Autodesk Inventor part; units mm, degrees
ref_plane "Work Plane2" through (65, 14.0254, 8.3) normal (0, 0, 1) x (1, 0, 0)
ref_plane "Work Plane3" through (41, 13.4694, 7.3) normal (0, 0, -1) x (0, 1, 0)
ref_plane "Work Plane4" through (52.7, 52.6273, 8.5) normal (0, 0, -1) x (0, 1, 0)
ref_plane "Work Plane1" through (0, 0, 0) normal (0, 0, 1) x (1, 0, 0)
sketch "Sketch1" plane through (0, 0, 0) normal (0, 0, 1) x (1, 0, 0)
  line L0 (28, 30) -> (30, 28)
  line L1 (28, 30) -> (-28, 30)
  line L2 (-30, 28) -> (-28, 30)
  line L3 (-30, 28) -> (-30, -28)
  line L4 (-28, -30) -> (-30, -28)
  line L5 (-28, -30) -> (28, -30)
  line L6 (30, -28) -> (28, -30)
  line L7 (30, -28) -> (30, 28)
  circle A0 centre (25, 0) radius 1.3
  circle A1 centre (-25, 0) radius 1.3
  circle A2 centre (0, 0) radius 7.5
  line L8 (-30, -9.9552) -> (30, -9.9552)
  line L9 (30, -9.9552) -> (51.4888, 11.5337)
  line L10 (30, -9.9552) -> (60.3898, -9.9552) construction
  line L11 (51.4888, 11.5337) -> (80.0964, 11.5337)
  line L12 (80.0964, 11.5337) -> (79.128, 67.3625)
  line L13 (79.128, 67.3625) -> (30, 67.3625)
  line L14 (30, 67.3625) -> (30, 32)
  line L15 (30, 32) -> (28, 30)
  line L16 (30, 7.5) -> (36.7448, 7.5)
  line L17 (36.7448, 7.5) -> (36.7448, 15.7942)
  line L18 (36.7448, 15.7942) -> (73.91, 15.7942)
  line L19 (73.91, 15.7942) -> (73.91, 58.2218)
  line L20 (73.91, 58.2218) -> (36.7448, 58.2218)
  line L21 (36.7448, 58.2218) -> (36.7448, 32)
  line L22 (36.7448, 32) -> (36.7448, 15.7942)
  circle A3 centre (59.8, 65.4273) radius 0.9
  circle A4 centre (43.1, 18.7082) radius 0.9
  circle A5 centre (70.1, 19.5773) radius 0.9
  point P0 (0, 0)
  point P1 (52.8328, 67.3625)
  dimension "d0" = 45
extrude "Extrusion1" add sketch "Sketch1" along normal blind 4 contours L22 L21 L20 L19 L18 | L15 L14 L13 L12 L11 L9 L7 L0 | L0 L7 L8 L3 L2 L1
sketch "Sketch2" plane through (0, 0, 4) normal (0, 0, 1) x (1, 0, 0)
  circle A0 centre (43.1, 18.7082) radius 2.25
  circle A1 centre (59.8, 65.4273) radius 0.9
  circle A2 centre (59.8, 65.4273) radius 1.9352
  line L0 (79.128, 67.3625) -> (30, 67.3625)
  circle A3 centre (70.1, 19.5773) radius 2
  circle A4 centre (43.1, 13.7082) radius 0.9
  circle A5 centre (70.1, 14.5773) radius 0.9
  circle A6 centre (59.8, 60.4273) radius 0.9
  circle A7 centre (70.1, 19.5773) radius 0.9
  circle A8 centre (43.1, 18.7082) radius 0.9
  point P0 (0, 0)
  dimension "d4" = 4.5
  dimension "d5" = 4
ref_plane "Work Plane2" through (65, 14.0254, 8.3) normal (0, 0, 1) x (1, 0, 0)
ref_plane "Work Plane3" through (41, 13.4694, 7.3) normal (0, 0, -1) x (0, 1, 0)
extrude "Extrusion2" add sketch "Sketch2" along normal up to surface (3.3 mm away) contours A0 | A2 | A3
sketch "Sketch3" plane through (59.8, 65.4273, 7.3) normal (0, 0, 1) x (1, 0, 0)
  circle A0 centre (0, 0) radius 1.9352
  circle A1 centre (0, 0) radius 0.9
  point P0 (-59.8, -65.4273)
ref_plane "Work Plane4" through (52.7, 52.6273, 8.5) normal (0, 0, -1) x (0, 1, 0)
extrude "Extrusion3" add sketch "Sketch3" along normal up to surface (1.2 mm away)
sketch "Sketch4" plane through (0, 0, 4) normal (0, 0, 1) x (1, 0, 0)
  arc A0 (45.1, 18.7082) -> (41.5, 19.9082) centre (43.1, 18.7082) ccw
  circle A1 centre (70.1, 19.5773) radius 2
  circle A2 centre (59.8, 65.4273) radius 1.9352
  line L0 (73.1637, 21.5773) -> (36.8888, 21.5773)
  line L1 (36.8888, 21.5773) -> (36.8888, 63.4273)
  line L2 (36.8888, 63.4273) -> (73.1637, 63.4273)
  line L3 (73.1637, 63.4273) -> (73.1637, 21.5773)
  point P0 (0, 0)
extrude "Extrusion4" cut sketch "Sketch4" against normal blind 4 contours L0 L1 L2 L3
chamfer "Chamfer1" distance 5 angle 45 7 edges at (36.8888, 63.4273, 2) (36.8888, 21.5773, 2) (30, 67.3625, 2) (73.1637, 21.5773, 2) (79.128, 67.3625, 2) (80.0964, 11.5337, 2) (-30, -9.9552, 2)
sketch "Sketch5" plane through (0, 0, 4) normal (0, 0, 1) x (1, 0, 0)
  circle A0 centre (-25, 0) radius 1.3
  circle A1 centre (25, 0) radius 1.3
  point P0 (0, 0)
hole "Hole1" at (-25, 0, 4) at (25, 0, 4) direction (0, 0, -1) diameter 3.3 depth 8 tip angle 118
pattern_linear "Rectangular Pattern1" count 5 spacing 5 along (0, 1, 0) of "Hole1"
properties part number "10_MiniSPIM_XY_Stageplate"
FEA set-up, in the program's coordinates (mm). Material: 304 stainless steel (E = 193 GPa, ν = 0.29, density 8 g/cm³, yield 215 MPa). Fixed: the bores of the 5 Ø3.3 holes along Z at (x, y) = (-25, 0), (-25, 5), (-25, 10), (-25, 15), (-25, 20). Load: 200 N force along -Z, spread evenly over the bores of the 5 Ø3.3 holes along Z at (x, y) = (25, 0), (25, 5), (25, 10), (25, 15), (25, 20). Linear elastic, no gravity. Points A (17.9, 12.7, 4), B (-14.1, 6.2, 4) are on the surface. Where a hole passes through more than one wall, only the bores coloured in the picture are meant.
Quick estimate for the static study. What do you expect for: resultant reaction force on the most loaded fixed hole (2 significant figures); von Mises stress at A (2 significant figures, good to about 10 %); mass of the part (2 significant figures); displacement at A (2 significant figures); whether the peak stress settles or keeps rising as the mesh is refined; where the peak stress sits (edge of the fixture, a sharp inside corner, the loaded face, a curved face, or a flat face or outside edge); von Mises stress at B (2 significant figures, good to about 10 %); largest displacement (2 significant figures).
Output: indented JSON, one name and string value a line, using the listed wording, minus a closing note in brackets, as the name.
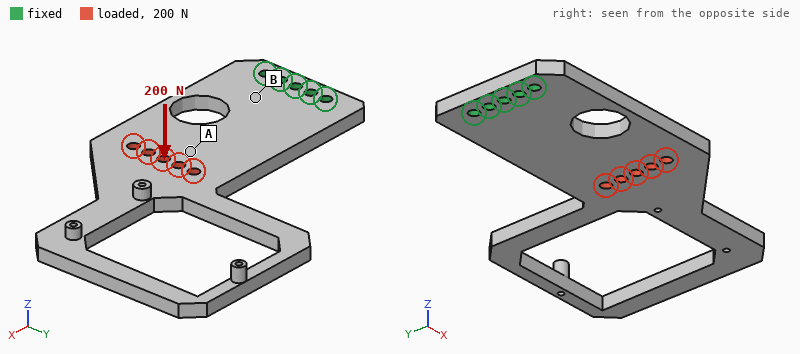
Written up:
{
  "resultant reaction force on the most loaded fixed hole": "89 N",
  "von Mises stress at A": "17 MPa",
  "mass of the part": "120 g",
  "displacement at A": "0.18 mm",
  "whether the peak stress settles or keeps rising as the mesh is refined": "keeps rising",
  "where the peak stress sits": "edge of the fixture",
  "von Mises stress at B": "67 MPa",
  "largest displacement": "0.62 mm"
}
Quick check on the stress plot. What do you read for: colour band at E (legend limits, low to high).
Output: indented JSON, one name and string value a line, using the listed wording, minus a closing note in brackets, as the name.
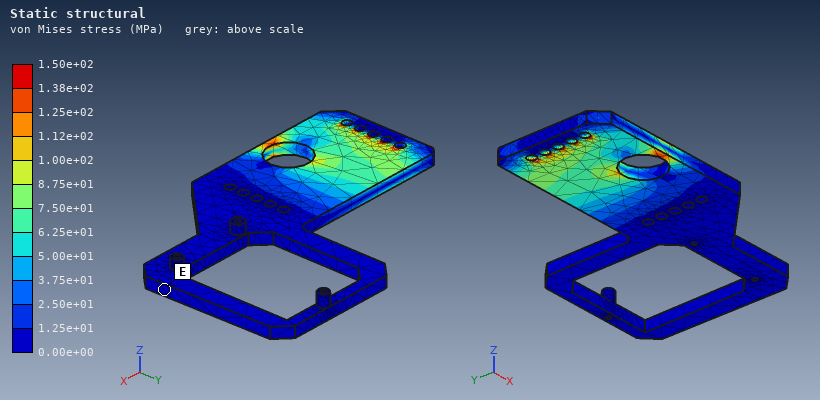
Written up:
{
  "colour band at E": "0.00e+00 to 1.25e+01 MPa"
}
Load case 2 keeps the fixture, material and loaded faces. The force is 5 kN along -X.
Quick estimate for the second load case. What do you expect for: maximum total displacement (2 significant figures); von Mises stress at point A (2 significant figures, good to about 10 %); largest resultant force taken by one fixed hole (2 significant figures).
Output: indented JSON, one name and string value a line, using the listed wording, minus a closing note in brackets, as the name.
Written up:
{
  "maximum total displacement": "28 µm",
  "von Mises stress at point A": "48 MPa",
  "largest resultant force taken by one fixed hole": "1.5 kN"
}
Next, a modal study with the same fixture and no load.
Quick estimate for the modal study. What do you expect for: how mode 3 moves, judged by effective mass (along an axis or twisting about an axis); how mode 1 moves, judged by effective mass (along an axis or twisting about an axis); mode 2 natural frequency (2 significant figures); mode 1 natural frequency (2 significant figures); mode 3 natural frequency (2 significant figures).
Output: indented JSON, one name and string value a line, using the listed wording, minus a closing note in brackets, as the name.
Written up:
{
  "how mode 3 moves, judged by effective mass": "along Z",
  "how mode 1 moves, judged by effective mass": "along Z",
  "mode 2 natural frequency": "830 Hz",
  "mode 1 natural frequency": "290 Hz",
  "mode 3 natural frequency": "1300 Hz"
}
